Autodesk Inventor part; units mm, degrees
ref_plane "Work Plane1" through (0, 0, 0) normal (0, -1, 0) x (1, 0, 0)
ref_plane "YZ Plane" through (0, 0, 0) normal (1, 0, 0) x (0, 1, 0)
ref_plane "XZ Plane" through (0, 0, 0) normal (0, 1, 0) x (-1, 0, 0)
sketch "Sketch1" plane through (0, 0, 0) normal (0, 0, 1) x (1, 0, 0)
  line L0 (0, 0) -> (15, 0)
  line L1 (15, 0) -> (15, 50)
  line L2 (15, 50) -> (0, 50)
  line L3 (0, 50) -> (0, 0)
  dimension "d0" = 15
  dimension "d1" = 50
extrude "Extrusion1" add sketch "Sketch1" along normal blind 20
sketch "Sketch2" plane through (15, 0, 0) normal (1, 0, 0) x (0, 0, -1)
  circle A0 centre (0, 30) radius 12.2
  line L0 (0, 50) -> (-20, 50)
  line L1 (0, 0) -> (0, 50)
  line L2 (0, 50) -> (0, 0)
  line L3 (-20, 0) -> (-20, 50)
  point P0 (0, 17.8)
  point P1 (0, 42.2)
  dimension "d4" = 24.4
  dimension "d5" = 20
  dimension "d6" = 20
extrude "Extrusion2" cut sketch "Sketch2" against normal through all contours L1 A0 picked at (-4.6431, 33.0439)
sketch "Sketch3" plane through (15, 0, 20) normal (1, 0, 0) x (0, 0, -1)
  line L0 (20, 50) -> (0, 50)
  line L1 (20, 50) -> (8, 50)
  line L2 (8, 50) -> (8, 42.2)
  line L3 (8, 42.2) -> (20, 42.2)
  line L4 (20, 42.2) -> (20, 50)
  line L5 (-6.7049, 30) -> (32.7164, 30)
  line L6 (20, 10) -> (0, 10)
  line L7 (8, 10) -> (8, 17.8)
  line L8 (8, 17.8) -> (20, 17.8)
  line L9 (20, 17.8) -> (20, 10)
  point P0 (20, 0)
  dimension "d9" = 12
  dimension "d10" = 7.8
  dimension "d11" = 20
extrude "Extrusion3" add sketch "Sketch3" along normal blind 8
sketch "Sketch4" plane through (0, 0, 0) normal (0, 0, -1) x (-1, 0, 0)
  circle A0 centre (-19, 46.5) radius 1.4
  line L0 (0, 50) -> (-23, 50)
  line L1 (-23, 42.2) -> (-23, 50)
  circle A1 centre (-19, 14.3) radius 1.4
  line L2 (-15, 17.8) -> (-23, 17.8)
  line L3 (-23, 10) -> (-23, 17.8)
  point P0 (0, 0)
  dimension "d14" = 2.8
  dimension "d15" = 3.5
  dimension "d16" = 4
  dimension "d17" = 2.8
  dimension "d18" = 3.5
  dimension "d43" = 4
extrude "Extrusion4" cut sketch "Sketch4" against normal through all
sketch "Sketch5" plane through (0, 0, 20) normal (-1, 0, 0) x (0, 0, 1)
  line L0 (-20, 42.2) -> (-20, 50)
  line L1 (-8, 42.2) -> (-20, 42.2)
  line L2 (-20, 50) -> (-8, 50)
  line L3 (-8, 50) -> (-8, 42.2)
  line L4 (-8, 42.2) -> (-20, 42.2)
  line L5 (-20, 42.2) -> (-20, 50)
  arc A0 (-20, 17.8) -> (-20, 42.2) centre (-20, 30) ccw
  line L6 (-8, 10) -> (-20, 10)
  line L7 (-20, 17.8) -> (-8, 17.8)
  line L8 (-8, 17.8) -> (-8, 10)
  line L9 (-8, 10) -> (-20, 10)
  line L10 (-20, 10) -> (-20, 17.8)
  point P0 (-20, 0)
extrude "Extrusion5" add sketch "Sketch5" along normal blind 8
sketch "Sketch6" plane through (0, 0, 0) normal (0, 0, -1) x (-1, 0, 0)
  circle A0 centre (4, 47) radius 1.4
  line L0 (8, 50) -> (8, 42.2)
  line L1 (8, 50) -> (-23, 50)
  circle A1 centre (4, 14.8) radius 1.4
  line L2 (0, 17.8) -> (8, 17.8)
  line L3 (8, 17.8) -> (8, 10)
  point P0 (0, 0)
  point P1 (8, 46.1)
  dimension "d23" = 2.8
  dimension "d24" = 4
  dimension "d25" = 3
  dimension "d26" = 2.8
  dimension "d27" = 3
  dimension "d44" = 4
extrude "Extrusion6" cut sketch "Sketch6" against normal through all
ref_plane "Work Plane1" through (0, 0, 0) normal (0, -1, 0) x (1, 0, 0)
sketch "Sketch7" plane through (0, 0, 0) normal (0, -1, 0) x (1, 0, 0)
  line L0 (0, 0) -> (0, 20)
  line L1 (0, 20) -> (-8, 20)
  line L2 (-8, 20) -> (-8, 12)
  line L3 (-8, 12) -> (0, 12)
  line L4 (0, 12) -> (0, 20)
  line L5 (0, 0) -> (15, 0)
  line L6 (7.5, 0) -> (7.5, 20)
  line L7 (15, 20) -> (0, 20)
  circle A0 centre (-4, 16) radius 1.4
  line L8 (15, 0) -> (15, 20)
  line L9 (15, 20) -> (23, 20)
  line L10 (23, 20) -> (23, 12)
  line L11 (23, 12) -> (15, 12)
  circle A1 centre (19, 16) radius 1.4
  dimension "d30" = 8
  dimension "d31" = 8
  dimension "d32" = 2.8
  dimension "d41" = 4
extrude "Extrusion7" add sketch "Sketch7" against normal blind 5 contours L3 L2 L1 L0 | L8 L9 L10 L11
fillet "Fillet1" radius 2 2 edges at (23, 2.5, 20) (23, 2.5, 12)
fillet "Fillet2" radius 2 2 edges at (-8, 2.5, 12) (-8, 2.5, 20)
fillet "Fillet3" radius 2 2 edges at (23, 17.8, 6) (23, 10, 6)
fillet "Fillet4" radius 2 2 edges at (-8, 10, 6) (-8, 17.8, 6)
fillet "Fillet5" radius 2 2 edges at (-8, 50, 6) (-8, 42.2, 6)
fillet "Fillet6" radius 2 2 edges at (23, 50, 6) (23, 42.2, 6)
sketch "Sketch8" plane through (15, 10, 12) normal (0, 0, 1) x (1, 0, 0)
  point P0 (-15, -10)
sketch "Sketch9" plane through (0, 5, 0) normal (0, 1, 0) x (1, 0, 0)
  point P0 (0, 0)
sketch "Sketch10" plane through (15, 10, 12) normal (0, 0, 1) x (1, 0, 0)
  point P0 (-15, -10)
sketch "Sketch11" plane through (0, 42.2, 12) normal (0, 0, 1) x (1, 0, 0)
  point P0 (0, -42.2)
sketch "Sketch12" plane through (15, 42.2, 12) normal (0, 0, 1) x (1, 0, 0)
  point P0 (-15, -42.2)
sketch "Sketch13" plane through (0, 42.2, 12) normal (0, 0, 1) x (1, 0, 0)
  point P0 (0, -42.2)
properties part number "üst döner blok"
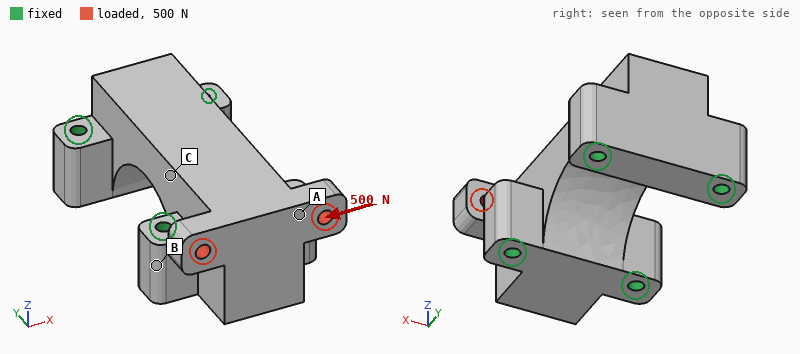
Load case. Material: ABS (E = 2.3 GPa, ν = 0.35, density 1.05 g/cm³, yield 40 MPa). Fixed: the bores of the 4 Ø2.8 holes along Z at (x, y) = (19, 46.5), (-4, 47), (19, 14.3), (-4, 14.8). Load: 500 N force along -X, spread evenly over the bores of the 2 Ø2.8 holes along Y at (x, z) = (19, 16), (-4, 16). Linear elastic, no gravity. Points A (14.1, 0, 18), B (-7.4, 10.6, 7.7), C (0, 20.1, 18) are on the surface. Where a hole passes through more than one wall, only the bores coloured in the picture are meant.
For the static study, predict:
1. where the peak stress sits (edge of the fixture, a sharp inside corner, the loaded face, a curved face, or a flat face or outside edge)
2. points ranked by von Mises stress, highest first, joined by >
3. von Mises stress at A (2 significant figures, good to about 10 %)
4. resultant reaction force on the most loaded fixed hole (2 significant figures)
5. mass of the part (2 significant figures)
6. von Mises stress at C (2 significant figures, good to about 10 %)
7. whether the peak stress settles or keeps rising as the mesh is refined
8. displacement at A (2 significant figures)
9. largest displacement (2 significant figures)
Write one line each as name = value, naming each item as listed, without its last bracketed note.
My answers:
where the peak stress sits = a sharp inside corner
points ranked by von Mises stress, highest first, joined by > = A > C > B
von Mises stress at A = 6.8 MPa
resultant reaction force on the most loaded fixed hole = 410 N
mass of the part = 15 g
von Mises stress at C = 3.0 MPa
whether the peak stress settles or keeps rising as the mesh is refined = keeps rising
displacement at A = 0.14 mm
largest displacement = 0.20 mm
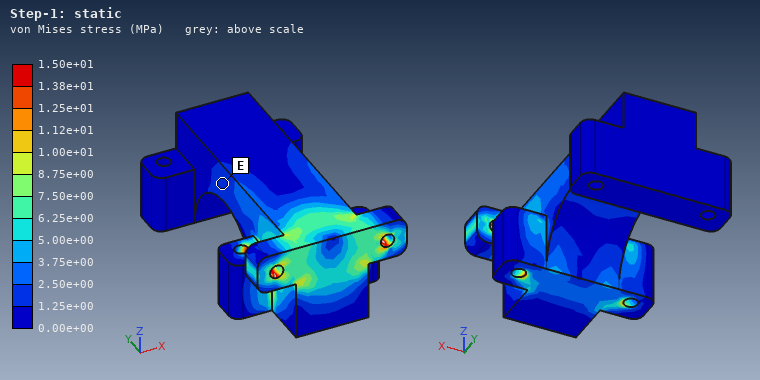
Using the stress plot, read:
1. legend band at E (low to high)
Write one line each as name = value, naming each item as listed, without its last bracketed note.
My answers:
legend band at E = 1.25e+00 to 2.50e+00 MPa
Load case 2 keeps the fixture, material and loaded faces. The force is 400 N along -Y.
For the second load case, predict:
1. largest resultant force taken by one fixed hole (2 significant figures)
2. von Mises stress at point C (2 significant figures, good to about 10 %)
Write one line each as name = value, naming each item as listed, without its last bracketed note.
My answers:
largest resultant force taken by one fixed hole = 130 N
von Mises stress at point C = 2.7 MPa
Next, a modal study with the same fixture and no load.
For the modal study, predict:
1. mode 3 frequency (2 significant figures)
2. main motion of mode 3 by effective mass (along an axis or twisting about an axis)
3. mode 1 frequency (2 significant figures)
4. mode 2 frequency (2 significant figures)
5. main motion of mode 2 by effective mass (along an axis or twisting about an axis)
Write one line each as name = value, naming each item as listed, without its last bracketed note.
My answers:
mode 3 frequency = 7800 Hz
main motion of mode 3 by effective mass = along Y
mode 1 frequency = 5100 Hz
mode 2 frequency = 6700 Hz
main motion of mode 2 by effective mass = along X
